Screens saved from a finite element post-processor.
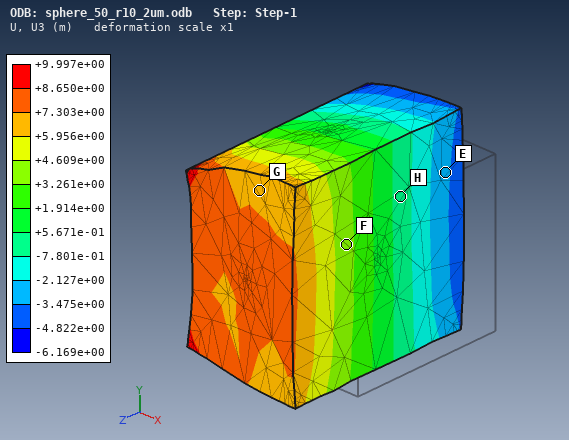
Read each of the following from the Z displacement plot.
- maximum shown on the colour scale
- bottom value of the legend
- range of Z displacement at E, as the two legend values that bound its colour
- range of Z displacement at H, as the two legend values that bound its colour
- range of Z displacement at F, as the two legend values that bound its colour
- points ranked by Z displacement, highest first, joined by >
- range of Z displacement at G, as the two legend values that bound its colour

+9.997e+00 m
-6.169e+00 m
-3.475e+00 to -2.127e+00 m
-7.801e-01 to +5.671e-01 m
+3.261e+00 to +4.609e+00 m
G > F > H > E
+5.956e+00 to +7.303e+00 m
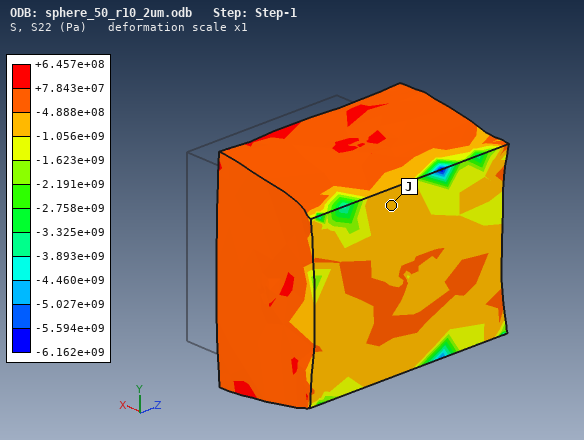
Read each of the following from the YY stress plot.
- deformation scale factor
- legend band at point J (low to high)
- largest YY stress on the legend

1
-1.056e+09 to -4.888e+08 Pa
+6.457e+08 Pa
